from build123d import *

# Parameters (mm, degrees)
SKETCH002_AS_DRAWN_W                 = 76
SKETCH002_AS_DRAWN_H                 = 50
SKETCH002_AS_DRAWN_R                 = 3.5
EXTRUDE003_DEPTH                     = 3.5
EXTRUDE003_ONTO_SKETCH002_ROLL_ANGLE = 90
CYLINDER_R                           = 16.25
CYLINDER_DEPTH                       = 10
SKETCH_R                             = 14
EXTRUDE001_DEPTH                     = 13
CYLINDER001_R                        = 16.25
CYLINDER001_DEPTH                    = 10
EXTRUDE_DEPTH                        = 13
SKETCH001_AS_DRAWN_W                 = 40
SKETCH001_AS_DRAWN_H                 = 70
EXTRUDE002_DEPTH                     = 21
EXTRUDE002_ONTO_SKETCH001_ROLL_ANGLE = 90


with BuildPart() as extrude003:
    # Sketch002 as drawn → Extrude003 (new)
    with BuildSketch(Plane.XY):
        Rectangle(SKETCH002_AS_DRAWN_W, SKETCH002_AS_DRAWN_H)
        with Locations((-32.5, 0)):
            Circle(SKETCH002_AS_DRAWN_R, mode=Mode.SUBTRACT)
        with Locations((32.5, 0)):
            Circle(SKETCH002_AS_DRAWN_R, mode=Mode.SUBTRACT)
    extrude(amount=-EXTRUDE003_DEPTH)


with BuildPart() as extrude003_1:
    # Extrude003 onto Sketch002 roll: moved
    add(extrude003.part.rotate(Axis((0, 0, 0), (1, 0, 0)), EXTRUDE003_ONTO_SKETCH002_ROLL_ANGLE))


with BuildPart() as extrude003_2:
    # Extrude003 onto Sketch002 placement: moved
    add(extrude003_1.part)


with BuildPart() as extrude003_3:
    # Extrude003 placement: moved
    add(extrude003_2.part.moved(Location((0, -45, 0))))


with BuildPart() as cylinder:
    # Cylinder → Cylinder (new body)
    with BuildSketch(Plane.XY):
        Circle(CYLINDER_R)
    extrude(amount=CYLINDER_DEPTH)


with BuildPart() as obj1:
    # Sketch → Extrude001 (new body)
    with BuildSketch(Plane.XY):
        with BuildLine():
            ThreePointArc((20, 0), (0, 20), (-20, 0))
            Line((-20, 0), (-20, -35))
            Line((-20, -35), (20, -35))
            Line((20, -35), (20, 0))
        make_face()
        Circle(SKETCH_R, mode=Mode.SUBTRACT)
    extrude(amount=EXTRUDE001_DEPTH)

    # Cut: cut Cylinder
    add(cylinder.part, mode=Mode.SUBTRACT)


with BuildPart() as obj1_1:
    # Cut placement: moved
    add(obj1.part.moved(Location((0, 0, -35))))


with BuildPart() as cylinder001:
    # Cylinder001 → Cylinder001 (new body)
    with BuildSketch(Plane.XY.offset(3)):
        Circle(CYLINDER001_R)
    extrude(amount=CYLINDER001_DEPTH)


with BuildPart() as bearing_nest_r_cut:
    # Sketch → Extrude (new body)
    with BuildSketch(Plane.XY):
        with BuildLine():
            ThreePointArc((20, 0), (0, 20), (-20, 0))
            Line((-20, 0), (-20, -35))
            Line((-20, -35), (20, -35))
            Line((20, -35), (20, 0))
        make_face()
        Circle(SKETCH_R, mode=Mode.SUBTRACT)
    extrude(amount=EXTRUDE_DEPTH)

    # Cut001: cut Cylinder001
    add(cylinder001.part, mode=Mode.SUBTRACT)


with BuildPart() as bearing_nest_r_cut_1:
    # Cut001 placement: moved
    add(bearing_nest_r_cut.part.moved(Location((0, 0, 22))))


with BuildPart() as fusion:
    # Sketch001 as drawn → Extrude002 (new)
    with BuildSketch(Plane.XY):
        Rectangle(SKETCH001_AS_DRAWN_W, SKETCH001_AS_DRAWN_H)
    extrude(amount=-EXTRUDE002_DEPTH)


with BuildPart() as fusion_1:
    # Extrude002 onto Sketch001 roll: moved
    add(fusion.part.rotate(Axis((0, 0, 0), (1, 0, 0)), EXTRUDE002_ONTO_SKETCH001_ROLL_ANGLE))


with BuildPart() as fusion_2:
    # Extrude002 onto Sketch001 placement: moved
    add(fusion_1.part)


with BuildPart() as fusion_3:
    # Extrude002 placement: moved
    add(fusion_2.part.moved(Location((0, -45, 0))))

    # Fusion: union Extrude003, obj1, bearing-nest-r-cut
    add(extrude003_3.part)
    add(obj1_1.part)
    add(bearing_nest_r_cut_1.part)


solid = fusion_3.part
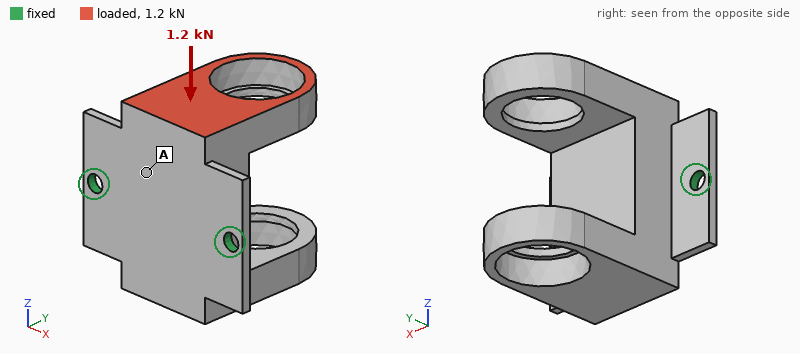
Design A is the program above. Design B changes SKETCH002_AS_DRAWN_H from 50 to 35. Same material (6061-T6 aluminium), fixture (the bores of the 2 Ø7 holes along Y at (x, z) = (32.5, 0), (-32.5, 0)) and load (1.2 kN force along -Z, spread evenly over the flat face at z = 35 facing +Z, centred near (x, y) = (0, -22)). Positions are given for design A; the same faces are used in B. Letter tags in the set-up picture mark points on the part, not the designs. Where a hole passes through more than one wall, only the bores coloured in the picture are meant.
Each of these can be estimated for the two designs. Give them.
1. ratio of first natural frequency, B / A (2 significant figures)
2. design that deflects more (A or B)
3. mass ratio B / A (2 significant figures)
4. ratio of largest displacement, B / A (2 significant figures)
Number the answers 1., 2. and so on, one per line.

1. 0.95
2. B
3. 0.98
4. 1.1
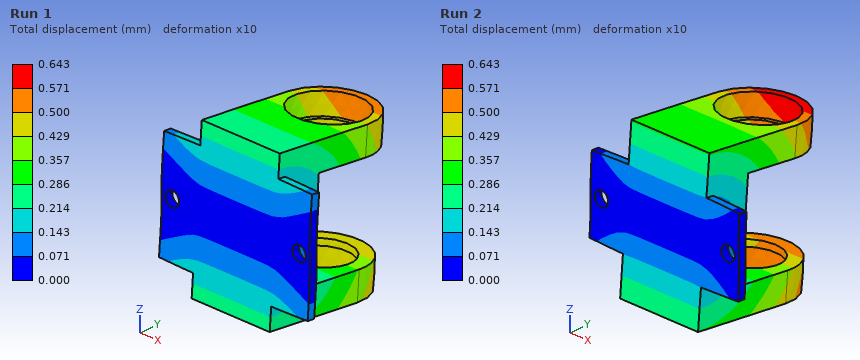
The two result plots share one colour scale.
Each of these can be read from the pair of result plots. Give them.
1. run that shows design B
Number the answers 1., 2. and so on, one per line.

1. Run 2
